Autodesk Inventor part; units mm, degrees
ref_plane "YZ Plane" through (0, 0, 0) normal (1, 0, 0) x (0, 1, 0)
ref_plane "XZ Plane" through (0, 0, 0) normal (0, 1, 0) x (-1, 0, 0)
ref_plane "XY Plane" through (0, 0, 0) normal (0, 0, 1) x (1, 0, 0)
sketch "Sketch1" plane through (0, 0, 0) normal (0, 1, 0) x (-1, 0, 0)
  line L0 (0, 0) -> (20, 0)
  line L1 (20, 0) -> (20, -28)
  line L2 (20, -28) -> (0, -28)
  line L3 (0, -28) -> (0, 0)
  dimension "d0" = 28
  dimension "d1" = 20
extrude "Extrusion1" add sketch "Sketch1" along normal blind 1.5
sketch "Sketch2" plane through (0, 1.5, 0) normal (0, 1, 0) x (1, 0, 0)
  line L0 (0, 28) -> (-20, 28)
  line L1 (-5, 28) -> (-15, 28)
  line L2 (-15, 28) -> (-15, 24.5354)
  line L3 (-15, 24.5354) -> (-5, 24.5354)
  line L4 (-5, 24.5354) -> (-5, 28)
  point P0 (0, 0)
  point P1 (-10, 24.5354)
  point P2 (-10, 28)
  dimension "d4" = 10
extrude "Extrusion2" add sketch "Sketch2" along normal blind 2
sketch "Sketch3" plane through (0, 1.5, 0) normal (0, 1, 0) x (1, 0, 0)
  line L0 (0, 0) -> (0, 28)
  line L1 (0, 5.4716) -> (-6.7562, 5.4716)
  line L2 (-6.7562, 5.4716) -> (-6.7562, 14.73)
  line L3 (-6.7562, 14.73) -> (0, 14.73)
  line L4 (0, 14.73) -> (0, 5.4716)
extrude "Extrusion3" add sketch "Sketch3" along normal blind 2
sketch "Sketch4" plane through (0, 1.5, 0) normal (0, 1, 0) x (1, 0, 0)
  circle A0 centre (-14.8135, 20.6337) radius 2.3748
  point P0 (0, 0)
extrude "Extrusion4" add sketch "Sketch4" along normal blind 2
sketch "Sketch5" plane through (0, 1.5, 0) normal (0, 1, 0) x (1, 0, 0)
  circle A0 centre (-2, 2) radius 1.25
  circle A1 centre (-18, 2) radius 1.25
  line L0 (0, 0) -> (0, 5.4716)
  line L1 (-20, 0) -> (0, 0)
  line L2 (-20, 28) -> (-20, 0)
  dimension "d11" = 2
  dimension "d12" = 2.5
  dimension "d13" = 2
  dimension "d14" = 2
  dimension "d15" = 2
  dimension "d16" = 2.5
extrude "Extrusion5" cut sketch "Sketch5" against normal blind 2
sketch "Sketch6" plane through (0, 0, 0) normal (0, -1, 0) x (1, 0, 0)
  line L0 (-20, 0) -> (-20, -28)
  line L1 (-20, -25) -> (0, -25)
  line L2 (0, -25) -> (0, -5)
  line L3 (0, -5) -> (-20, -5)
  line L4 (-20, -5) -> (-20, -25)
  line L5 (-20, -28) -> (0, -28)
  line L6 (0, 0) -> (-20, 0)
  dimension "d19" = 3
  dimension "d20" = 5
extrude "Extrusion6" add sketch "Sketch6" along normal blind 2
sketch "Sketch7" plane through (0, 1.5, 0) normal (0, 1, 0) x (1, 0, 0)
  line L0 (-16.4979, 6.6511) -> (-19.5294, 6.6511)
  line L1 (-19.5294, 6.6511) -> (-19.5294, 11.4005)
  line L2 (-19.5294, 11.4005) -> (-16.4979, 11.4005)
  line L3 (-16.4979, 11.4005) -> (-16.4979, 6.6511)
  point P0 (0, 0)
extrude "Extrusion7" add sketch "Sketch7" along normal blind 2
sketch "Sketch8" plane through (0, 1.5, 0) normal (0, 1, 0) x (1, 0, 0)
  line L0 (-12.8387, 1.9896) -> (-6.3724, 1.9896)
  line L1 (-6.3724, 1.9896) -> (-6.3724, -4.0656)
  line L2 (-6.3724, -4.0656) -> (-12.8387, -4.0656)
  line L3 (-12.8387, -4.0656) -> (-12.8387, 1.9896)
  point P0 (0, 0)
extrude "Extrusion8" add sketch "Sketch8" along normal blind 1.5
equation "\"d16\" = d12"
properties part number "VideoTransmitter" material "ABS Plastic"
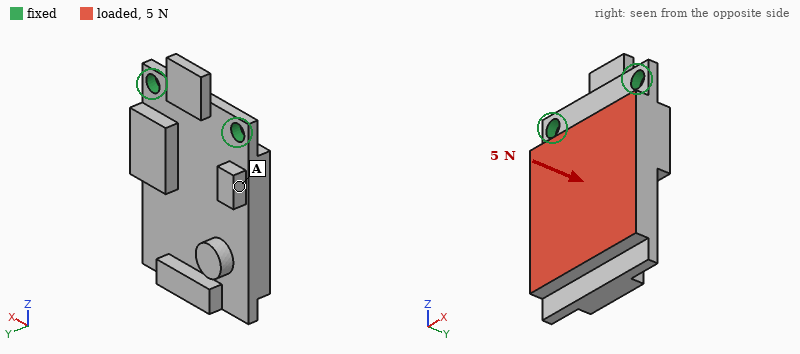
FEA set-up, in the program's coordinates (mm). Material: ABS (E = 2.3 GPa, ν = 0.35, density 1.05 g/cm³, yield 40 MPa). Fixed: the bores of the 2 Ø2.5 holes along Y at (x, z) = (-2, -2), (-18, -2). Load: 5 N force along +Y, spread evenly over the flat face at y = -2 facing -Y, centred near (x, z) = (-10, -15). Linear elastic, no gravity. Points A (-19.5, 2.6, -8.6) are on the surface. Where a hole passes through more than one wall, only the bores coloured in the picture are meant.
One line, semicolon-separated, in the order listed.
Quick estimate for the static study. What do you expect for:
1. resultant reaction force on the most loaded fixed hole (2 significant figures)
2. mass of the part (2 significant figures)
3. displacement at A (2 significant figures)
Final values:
2.8 N; 2.0 g; 0.076 mm
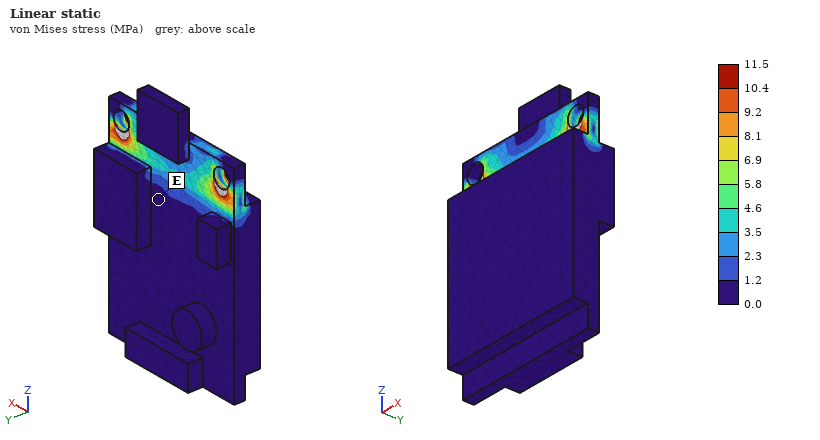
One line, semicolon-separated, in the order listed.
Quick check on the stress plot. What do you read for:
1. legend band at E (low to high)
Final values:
0.0 to 1.2 MPa
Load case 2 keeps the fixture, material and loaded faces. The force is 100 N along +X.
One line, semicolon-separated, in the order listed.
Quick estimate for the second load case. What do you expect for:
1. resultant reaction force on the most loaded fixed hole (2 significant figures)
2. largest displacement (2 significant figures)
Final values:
93 N; 0.13 mm
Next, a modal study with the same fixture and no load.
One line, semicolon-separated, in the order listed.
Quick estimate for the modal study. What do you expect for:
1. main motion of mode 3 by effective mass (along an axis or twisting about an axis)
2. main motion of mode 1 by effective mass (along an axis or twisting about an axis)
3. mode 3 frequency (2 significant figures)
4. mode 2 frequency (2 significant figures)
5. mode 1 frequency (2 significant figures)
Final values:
along X; along Y; 4500 Hz; 3000 Hz; 510 Hz
